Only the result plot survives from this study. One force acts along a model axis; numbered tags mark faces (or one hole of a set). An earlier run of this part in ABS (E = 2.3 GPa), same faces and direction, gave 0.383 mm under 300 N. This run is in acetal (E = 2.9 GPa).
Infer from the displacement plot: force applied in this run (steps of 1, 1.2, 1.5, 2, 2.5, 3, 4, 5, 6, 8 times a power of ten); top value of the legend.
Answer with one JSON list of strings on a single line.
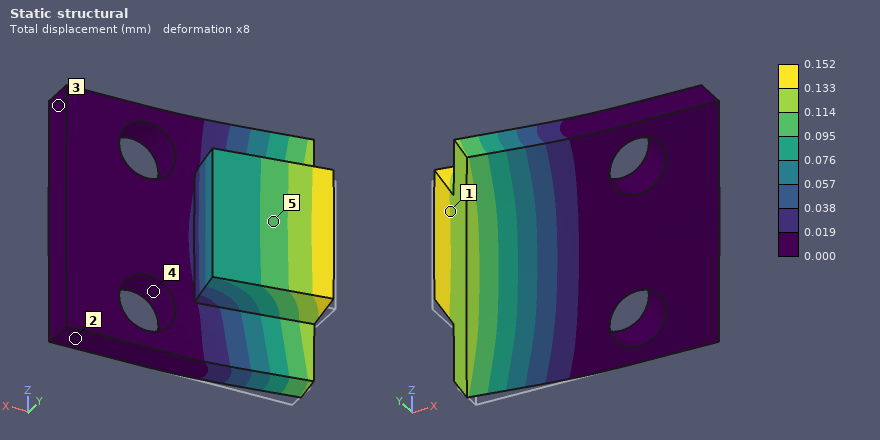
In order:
["150 N", "0.152 mm"]
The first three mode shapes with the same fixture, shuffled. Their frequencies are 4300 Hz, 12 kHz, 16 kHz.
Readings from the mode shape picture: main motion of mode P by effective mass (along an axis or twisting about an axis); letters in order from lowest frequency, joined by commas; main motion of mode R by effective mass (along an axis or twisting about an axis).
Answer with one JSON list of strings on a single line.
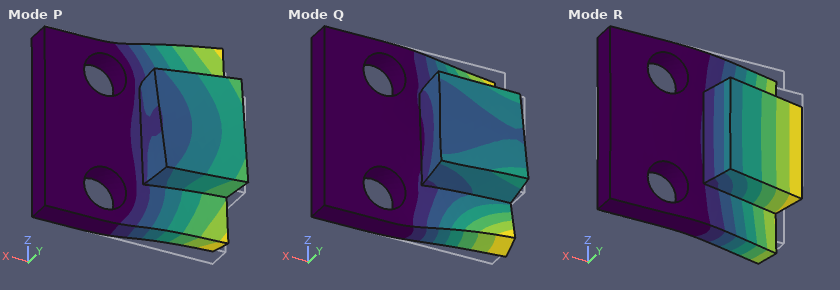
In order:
["along Z", "R, Q, P", "along Y"]
